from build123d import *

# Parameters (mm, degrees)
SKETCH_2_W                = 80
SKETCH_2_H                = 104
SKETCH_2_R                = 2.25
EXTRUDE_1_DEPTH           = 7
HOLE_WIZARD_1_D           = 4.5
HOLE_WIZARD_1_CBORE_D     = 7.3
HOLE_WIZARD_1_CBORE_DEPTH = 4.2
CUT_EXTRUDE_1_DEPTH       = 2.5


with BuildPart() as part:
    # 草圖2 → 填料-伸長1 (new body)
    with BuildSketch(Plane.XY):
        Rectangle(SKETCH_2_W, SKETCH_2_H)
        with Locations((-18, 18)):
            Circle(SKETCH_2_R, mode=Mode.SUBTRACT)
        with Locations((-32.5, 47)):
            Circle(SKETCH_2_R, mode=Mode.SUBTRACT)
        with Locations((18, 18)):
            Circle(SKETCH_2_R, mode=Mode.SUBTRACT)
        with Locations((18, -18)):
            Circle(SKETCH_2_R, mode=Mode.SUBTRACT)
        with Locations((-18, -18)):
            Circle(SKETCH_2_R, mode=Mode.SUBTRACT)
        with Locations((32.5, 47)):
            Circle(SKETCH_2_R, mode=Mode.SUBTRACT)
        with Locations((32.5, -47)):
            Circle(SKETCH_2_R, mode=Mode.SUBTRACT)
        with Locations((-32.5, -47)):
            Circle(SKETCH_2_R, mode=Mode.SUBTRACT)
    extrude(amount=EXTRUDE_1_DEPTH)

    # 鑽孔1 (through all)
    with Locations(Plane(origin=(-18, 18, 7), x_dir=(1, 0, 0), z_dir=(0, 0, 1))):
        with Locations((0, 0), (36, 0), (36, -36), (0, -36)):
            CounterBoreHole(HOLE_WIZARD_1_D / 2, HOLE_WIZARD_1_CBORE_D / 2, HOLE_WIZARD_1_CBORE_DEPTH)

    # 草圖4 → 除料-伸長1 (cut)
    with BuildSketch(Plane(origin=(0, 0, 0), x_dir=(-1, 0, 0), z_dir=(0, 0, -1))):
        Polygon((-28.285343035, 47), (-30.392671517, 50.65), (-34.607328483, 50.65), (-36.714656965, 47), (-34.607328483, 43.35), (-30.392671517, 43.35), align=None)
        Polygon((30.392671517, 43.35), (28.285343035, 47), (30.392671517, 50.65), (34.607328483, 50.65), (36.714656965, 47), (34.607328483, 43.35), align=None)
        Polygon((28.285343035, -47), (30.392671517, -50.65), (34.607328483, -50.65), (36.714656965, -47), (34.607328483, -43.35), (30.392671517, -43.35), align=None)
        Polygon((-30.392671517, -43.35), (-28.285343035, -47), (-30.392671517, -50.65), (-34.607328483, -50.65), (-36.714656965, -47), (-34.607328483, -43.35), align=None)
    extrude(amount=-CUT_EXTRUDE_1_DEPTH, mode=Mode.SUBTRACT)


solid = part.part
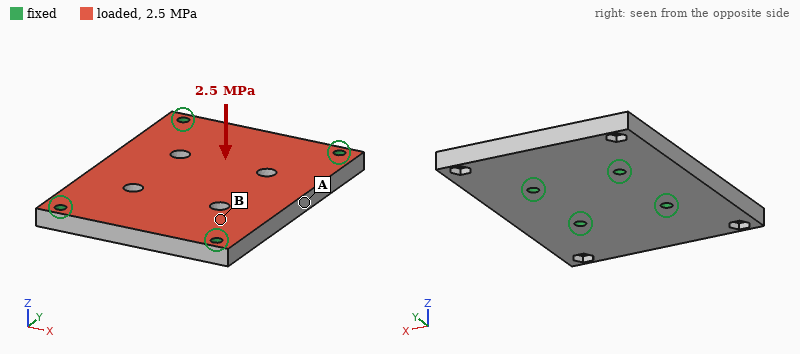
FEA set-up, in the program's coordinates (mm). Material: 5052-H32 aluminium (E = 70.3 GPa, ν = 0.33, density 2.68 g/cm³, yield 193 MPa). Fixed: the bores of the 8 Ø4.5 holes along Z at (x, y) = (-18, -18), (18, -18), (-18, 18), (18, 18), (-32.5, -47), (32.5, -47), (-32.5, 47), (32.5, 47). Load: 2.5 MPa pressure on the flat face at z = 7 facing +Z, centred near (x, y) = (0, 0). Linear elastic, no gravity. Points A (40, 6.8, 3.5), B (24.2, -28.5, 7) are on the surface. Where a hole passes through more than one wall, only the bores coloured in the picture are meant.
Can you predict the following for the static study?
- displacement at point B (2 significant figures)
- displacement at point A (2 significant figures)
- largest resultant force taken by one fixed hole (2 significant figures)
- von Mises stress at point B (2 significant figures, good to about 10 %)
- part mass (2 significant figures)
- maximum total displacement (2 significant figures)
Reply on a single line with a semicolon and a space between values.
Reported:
16 µm; 47 µm; 3.3 kN; 47 MPa; 150 g; 60 µm
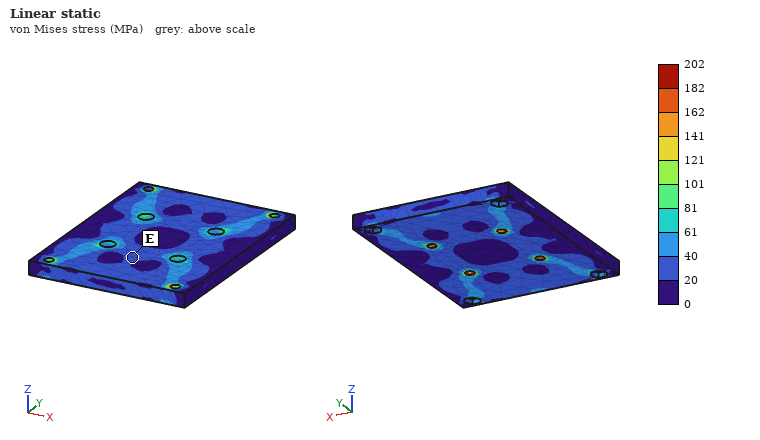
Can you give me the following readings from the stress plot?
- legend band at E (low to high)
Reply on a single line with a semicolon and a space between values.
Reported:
20 to 40 MPa
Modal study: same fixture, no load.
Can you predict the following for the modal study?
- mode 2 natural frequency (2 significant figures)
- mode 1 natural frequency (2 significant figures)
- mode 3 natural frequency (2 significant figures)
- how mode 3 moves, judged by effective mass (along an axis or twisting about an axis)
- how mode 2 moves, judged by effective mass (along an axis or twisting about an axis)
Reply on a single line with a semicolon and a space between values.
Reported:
8700 Hz; 7700 Hz; 9200 Hz; twisting about Y; twisting about X
